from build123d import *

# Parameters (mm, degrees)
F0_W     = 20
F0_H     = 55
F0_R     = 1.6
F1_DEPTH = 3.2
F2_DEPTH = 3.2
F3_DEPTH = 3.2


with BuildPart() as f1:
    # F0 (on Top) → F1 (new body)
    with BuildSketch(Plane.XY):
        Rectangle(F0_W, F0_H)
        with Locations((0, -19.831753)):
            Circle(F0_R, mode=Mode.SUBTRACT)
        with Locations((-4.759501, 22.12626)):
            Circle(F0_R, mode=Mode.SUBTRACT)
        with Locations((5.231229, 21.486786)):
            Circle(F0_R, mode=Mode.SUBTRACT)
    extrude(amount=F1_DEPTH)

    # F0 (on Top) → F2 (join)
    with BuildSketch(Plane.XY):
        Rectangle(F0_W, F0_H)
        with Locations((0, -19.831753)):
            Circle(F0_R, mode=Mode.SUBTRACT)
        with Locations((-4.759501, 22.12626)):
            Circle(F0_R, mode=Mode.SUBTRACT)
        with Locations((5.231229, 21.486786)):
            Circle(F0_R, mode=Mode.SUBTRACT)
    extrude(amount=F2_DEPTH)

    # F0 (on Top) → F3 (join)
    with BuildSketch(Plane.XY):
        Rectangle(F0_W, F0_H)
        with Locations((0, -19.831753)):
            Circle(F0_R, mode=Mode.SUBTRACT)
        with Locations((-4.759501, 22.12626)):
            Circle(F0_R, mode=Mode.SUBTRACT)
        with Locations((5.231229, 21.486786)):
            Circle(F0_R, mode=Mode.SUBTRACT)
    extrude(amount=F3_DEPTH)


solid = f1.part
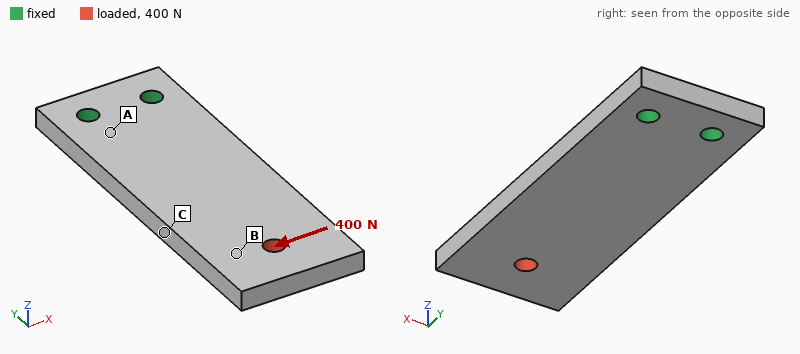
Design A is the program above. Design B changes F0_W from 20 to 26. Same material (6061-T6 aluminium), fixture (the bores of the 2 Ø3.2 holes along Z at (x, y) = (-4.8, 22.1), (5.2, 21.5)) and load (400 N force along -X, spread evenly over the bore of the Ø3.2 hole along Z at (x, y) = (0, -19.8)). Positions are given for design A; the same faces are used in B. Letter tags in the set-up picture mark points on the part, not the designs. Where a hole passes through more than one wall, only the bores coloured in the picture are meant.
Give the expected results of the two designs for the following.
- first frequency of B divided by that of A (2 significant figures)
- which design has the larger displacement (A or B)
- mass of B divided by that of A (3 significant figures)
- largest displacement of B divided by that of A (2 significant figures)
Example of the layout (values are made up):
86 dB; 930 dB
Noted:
0.99; A; 1.31; 0.68
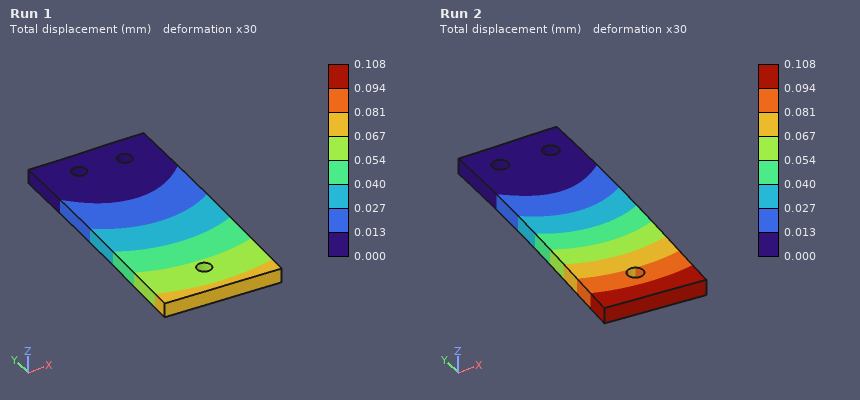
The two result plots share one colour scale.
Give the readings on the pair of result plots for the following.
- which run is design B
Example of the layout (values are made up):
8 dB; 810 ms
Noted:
Run 1
